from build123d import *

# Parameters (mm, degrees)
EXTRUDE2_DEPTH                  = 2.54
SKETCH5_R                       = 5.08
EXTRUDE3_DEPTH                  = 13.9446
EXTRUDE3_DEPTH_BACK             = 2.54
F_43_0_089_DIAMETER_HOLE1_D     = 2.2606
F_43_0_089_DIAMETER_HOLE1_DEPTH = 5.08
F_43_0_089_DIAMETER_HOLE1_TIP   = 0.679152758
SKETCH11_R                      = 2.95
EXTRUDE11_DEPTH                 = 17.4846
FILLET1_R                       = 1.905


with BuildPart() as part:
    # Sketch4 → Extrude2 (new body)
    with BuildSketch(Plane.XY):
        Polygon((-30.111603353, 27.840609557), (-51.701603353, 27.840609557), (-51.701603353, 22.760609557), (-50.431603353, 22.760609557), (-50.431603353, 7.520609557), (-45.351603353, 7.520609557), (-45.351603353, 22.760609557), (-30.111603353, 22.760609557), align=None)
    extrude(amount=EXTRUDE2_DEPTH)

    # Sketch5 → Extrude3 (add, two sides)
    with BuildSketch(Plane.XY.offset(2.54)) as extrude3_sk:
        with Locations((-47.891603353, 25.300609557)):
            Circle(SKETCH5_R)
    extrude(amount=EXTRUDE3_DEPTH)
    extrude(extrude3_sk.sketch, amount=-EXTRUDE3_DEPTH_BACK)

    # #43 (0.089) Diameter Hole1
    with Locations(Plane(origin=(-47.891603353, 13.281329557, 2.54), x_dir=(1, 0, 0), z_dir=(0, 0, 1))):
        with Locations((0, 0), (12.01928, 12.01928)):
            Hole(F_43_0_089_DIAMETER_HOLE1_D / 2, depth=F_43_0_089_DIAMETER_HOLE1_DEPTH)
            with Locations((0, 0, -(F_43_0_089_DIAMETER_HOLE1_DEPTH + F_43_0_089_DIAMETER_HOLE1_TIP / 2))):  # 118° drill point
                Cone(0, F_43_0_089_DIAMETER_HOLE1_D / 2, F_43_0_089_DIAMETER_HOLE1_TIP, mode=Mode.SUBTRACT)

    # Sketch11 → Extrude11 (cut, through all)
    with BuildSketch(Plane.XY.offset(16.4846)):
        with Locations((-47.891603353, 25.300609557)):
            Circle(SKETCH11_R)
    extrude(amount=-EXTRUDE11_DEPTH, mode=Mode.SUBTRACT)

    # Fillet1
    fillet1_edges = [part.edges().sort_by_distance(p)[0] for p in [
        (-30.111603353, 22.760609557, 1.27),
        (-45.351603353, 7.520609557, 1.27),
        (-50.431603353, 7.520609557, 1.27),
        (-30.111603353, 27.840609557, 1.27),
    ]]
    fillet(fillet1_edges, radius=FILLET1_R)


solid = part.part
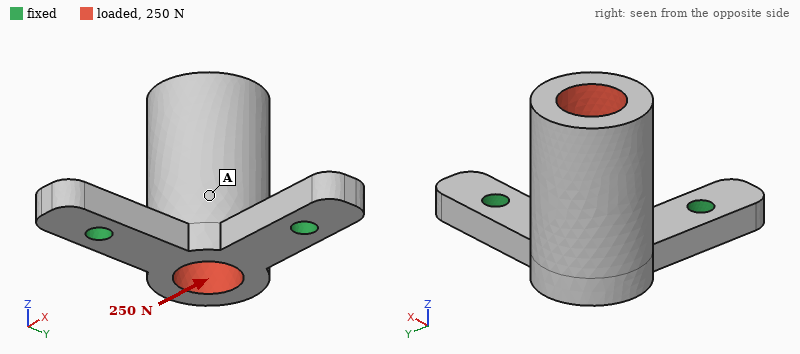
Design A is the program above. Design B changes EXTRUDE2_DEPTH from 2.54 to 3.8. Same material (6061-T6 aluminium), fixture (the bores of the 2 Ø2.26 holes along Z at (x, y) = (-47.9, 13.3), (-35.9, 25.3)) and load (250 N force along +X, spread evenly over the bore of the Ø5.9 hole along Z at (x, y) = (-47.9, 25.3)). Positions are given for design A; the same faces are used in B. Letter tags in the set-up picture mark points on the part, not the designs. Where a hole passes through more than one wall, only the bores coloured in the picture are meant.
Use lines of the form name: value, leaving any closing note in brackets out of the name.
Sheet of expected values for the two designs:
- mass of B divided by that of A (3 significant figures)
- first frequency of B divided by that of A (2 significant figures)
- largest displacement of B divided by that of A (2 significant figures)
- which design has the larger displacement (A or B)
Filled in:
mass of B divided by that of A: 1.13
first frequency of B divided by that of A: 1.7
largest displacement of B divided by that of A: 0.35
which design has the larger displacement: A
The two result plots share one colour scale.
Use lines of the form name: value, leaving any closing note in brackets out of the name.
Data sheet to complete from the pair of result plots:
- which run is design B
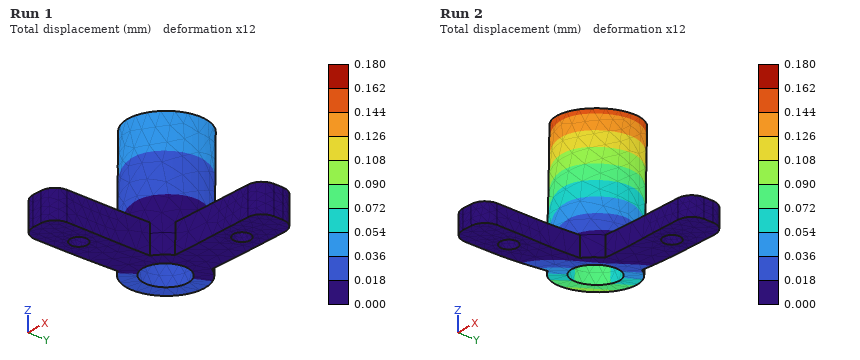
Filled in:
which run is design B: Run 1
